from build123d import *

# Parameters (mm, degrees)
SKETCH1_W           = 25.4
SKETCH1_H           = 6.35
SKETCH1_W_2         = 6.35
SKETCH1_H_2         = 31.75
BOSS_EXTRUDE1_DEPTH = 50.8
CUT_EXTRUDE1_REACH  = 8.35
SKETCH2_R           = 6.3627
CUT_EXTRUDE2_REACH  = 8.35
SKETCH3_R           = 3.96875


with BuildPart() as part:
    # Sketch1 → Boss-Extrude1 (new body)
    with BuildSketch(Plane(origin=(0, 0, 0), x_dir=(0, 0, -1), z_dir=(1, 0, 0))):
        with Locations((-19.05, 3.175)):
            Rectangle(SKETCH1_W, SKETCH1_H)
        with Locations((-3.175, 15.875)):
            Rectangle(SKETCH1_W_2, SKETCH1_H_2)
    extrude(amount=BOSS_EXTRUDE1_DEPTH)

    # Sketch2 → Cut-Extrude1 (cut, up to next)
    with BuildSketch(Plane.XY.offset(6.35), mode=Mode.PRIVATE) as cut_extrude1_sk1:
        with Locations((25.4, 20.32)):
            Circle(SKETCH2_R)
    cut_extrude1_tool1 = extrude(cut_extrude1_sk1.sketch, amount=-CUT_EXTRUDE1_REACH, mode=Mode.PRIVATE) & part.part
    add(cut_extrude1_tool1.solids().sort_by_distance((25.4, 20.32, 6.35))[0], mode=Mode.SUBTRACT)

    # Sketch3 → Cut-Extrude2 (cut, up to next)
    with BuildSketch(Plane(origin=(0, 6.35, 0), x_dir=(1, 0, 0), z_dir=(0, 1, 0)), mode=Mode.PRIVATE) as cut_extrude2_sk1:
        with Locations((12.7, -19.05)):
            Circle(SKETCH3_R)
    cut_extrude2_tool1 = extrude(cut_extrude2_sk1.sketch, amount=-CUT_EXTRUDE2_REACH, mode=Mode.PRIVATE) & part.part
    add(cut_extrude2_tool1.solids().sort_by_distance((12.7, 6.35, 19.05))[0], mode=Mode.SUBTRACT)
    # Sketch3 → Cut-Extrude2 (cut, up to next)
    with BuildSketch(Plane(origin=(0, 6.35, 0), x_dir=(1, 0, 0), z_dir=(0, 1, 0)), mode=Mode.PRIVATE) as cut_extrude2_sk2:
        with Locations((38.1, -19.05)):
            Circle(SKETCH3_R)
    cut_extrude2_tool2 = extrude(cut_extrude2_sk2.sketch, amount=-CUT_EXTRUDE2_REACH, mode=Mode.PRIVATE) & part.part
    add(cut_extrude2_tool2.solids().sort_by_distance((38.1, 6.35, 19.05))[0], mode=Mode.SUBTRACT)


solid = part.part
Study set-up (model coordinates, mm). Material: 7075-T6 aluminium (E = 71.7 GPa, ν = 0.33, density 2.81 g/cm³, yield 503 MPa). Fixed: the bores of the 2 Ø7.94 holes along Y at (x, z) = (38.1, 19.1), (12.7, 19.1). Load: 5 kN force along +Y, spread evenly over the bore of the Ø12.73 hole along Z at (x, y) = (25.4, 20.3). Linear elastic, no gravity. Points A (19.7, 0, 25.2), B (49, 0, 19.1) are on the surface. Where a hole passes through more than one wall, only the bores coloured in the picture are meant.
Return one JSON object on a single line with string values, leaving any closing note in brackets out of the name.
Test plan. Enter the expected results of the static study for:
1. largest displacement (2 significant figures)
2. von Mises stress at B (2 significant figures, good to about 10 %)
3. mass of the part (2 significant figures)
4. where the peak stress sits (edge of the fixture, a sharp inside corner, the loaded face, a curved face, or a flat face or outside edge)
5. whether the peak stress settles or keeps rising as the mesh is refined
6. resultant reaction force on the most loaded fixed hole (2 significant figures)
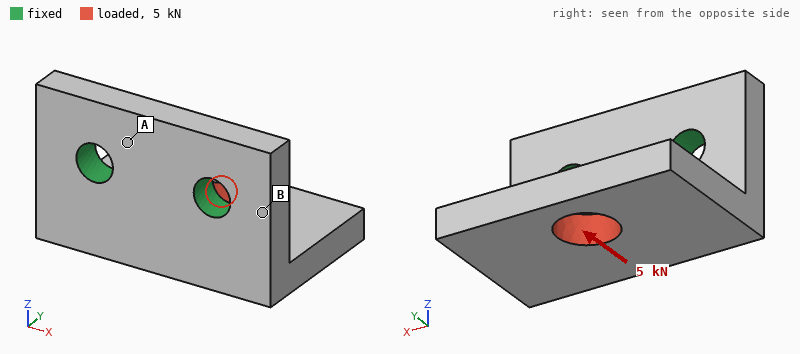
{"largest displacement": "0.21 mm", "von Mises stress at B": "61 MPa", "mass of the part": "48 g", "where the peak stress sits": "edge of the fixture", "whether the peak stress settles or keeps rising as the mesh is refined": "keeps rising", "resultant reaction force on the most loaded fixed hole": "2.5 kN"}
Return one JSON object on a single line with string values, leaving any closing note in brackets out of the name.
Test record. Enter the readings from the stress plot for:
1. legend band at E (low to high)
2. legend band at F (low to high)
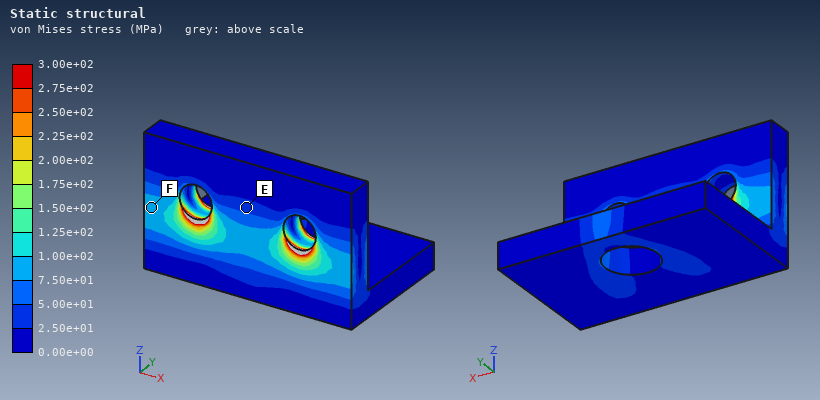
{"legend band at E": "2.50e+01 to 5.00e+01 MPa", "legend band at F": "7.50e+01 to 1.00e+02 MPa"}
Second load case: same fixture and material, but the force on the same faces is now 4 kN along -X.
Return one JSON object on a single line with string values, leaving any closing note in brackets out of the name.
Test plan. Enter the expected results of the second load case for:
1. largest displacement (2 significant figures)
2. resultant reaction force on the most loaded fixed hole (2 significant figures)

{"largest displacement": "0.12 mm", "resultant reaction force on the most loaded fixed hole": "3.4 kN"}
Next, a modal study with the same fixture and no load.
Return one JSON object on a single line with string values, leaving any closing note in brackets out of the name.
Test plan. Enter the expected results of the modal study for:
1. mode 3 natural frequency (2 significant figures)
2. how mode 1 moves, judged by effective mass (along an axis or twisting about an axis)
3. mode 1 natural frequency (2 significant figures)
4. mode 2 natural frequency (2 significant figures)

{"mode 3 natural frequency": "9200 Hz", "how mode 1 moves, judged by effective mass": "along Z", "mode 1 natural frequency": "3800 Hz", "mode 2 natural frequency": "6200 Hz"}
